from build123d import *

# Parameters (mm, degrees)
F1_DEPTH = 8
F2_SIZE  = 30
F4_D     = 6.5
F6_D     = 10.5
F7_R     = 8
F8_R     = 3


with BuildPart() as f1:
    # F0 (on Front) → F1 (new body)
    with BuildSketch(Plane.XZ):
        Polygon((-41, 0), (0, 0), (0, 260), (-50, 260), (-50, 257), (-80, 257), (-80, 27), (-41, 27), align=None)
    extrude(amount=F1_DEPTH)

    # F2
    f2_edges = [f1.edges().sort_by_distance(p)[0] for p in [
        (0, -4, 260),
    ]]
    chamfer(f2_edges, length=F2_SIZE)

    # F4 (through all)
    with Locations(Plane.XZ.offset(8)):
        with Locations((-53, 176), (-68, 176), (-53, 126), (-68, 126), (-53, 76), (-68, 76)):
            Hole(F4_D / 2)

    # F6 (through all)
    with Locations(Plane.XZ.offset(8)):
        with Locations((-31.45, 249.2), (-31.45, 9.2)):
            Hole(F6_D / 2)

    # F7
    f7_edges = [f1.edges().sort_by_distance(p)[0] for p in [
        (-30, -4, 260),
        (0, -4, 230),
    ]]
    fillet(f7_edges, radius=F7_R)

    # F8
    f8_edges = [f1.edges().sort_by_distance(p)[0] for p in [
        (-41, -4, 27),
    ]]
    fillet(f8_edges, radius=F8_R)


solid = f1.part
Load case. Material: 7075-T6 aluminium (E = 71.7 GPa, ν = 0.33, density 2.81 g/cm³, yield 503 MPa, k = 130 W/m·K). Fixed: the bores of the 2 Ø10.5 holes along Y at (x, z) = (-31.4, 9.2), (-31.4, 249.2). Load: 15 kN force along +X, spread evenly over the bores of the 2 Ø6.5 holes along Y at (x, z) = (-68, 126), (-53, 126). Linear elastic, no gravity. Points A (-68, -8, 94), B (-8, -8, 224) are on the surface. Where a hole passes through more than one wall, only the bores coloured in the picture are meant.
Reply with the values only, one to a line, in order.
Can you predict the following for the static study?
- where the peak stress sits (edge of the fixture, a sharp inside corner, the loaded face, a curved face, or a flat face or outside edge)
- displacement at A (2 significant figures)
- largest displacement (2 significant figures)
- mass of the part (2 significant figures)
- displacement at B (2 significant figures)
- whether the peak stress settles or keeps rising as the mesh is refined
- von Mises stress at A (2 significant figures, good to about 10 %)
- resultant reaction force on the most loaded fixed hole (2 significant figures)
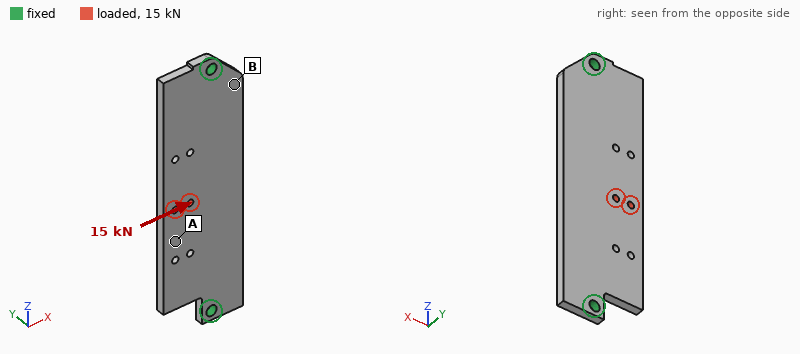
edge of the fixture
0.18 mm
0.22 mm
420 g
0.073 mm
keeps rising
45 MPa
8.4 kN
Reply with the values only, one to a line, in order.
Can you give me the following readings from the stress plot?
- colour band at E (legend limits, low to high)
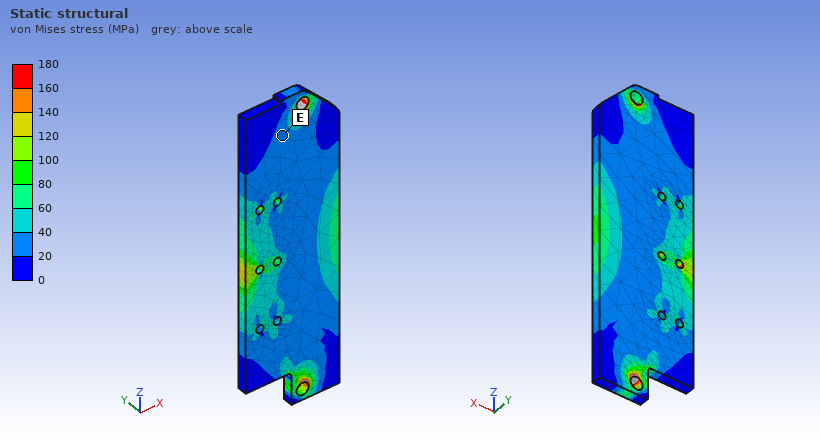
20 to 40 MPa
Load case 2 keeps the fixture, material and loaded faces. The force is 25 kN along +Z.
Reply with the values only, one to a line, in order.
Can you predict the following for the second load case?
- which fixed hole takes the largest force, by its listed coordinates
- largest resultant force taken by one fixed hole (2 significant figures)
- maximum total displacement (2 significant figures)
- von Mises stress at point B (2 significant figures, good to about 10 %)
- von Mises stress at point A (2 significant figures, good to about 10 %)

(-31.4, 249.2)
14 kN
76 µm
14 MPa
27 MPa
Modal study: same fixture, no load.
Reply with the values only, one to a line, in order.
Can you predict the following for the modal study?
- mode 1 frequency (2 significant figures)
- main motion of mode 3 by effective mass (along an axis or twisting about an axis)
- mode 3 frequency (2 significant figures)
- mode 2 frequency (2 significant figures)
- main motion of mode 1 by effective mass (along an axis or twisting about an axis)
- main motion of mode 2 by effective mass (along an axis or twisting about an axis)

610 Hz
twisting about X
1700 Hz
1100 Hz
along Y
twisting about Z
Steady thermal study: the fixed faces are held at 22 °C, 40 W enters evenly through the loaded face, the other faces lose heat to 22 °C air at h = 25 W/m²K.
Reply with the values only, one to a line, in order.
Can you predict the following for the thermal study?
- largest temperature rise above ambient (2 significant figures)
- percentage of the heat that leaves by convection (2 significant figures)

35 K
38 %
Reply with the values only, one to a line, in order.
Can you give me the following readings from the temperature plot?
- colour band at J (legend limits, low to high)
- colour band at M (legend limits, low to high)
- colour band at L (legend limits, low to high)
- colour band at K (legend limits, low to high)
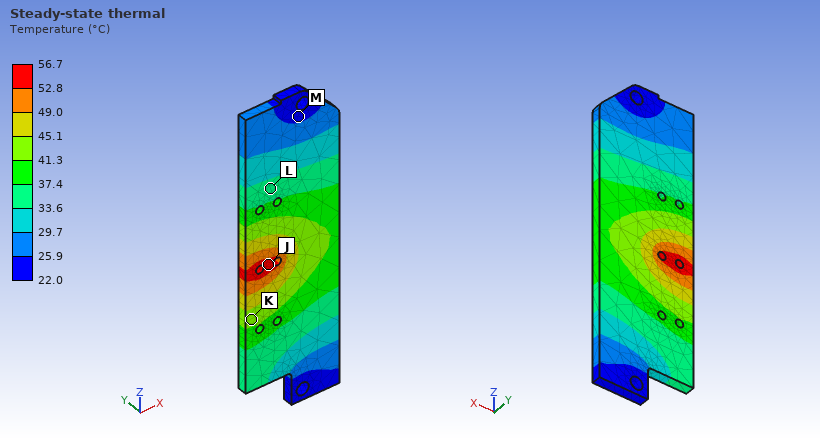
52.8 to 56.7 °C
22.0 to 25.9 °C
33.6 to 37.4 °C
41.3 to 45.1 °C
